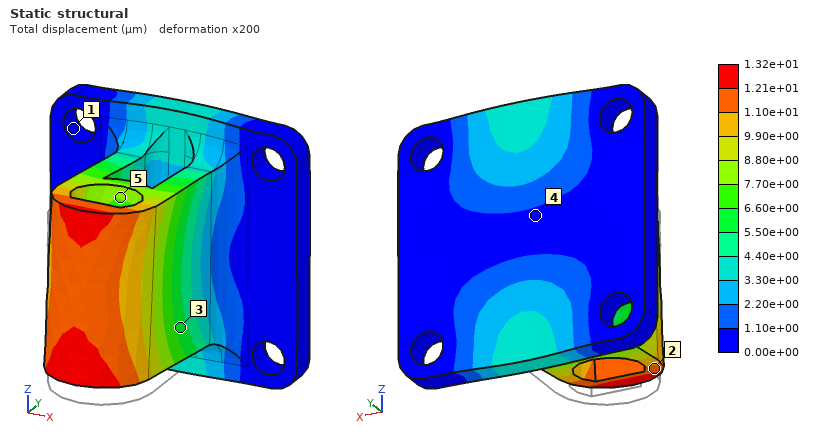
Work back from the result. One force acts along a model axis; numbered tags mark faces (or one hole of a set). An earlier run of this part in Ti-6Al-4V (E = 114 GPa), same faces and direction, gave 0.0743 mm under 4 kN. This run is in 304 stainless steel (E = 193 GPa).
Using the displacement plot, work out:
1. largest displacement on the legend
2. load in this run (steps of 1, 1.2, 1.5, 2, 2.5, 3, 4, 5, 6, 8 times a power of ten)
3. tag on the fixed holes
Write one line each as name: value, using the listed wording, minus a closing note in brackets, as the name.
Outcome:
largest displacement on the legend: 1.32e+01 µm
load in this run: 1.2 kN
tag on the fixed holes: 1
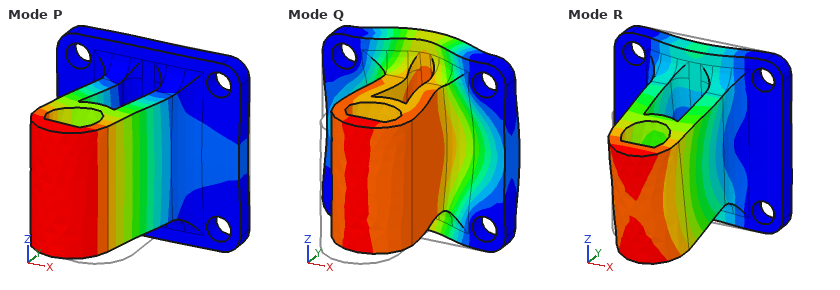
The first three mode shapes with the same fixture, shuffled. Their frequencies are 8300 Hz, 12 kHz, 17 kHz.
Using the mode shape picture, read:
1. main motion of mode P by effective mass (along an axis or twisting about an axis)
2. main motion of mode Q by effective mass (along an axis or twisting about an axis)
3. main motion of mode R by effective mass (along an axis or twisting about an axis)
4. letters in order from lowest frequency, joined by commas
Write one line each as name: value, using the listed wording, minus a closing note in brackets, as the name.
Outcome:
main motion of mode P by effective mass: along X
main motion of mode Q by effective mass: along Y
main motion of mode R by effective mass: along Z
letters in order from lowest frequency, joined by commas: P, R, Q
